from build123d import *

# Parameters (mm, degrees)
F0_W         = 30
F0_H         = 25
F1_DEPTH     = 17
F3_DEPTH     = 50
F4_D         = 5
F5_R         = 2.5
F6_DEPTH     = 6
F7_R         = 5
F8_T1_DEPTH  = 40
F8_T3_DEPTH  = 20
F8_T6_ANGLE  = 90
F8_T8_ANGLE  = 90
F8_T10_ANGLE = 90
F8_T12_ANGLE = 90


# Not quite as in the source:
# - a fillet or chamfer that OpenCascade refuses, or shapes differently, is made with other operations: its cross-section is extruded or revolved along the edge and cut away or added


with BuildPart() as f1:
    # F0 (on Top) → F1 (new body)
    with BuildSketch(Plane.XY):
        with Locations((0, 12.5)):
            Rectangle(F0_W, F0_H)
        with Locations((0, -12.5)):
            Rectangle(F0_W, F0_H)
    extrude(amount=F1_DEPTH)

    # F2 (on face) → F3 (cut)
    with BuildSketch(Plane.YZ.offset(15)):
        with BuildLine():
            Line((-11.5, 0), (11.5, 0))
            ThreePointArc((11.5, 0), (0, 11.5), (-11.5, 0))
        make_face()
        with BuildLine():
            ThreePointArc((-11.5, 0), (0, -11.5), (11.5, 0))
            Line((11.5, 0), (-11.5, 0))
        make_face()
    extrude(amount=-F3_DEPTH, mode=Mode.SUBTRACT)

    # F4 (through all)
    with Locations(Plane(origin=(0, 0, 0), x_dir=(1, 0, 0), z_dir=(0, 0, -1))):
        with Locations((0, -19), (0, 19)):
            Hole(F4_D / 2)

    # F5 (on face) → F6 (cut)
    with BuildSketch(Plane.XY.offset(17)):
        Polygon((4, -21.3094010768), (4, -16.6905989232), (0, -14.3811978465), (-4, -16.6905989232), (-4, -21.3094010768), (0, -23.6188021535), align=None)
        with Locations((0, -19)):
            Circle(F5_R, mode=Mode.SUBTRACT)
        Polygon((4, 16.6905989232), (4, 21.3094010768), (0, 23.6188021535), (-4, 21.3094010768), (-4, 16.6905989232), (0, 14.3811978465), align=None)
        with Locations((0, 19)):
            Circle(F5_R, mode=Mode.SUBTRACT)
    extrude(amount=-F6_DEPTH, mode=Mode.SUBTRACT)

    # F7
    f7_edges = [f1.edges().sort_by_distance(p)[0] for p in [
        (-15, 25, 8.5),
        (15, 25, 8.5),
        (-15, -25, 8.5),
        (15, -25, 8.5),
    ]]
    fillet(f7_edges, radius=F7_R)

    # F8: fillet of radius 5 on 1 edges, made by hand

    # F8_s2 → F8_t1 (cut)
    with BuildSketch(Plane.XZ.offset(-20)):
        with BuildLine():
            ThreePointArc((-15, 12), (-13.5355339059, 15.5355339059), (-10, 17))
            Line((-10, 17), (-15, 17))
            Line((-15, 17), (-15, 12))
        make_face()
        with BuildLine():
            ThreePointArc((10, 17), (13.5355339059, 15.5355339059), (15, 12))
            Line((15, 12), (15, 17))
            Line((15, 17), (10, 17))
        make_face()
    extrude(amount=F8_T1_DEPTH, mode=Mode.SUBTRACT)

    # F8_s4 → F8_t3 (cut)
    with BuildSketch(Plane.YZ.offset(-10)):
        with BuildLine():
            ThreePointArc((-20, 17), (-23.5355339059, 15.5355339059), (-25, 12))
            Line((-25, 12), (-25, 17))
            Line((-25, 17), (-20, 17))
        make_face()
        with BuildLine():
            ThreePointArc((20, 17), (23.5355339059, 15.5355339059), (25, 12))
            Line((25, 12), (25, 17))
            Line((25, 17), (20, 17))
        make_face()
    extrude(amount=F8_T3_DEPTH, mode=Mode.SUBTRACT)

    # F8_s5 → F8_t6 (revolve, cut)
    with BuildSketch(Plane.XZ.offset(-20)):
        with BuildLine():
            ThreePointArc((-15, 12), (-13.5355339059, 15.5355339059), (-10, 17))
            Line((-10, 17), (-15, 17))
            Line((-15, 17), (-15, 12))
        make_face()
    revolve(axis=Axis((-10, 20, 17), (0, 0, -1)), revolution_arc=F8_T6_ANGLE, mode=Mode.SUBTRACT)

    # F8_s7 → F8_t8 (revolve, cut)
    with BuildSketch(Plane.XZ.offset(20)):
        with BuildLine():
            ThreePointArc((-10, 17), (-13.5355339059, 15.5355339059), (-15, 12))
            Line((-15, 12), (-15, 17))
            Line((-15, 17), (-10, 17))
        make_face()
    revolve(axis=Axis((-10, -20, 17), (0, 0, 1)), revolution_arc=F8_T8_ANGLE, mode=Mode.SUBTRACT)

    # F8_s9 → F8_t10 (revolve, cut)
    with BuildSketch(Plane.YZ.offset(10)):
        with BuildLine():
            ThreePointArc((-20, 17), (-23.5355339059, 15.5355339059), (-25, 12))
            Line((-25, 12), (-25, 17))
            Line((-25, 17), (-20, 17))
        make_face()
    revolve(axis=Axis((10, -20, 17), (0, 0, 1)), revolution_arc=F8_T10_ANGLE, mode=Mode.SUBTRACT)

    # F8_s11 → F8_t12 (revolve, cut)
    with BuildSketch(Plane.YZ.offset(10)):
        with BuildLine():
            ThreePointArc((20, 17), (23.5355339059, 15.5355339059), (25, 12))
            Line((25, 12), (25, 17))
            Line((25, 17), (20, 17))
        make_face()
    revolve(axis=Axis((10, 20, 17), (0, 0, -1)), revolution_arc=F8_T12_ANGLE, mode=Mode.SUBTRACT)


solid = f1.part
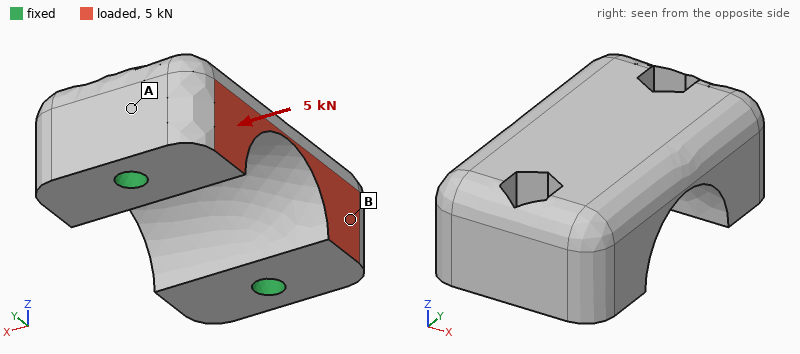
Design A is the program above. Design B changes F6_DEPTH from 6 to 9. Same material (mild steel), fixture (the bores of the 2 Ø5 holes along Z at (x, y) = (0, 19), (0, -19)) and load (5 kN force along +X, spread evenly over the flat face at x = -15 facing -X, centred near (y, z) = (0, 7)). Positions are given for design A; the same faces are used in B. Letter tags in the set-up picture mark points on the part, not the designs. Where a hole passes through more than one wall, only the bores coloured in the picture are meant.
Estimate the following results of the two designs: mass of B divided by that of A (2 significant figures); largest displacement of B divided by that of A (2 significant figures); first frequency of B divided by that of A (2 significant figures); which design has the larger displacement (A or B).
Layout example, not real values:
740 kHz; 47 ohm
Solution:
0.99; 1.7; 0.70; B
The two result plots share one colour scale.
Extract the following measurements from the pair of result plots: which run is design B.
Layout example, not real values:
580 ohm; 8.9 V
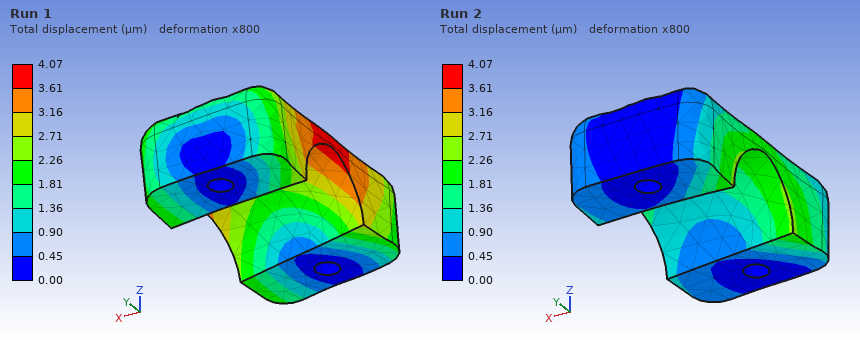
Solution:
Run 1
